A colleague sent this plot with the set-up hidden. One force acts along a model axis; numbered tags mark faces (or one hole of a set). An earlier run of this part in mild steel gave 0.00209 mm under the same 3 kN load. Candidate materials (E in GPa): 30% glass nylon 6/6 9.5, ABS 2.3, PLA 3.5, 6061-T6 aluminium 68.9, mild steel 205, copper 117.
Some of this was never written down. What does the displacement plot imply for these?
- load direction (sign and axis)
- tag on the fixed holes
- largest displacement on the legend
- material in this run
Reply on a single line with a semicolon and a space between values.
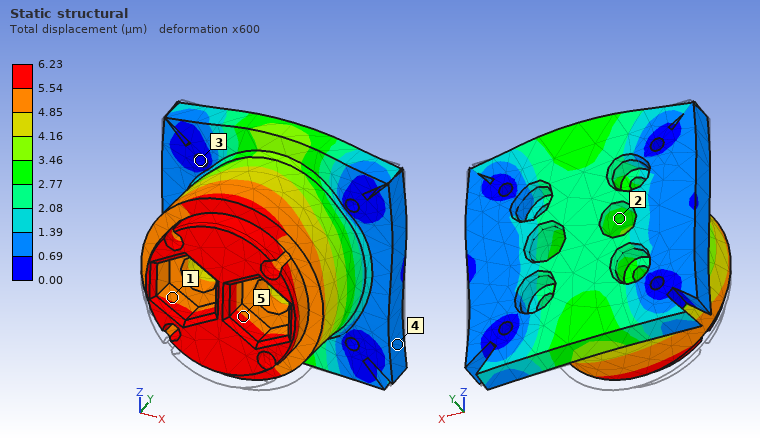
+Z; 3; 6.23 µm; 6061-T6 aluminium
